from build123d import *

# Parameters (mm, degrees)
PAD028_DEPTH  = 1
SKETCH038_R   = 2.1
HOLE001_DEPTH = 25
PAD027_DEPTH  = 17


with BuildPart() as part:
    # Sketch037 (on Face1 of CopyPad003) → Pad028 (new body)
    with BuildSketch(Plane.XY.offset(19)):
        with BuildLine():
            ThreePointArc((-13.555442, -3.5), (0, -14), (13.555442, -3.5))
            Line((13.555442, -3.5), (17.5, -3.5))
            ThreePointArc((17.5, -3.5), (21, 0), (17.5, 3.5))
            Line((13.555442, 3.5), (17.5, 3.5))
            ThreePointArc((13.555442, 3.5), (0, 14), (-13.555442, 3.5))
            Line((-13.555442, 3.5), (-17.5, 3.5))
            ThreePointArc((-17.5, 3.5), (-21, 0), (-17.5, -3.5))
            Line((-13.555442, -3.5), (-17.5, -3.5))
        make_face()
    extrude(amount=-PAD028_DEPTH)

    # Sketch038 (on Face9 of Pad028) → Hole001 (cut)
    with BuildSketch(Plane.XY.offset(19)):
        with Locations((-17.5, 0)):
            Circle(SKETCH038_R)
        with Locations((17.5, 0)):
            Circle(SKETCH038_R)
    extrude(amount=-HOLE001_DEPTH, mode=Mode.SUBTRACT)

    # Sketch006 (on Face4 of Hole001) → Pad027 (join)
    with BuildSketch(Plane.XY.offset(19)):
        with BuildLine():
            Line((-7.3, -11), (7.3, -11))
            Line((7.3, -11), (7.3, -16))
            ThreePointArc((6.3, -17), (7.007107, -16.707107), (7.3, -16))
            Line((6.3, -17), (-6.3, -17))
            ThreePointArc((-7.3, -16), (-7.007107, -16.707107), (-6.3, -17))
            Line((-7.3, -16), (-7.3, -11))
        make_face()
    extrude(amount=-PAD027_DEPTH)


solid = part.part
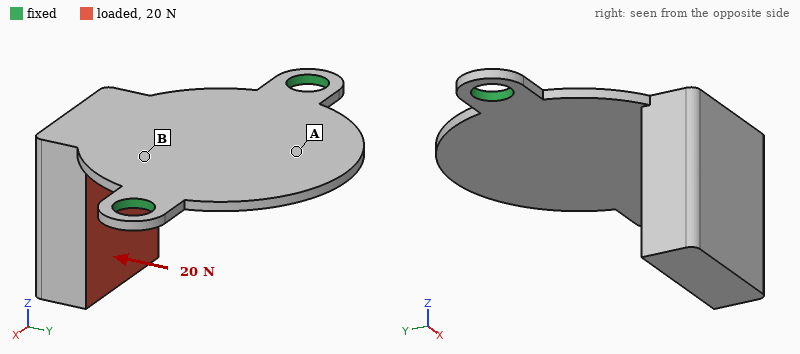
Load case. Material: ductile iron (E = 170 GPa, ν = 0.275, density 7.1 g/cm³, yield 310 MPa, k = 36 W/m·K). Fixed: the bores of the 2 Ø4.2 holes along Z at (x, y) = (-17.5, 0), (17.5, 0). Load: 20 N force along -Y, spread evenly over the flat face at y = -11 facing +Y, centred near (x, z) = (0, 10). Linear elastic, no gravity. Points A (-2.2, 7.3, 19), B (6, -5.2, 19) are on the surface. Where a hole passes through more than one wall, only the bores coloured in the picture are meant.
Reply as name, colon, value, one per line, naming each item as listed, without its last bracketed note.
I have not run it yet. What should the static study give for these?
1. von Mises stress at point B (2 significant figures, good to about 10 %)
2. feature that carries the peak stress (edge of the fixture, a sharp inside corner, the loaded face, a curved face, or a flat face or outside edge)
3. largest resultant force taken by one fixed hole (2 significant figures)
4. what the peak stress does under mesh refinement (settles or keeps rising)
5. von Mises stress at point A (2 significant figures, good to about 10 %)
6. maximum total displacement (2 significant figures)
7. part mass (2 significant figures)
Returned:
von Mises stress at point B: 36 MPa
feature that carries the peak stress: a sharp inside corner
largest resultant force taken by one fixed hole: 10 N
what the peak stress does under mesh refinement: keeps rising
von Mises stress at point A: 8.2 MPa
maximum total displacement: 0.16 mm
part mass: 15 g
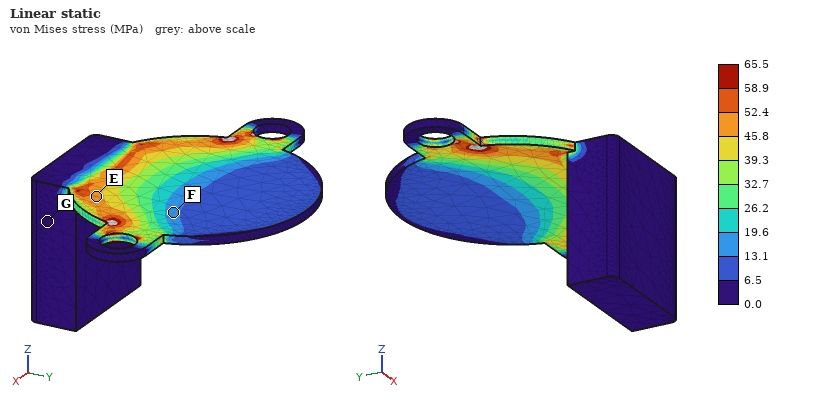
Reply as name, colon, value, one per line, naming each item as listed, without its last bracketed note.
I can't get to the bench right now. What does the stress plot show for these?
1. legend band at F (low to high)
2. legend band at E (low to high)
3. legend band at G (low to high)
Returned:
legend band at F: 13.1 to 19.6 MPa
legend band at E: 45.8 to 52.4 MPa
legend band at G: 0.0 to 6.5 MPa
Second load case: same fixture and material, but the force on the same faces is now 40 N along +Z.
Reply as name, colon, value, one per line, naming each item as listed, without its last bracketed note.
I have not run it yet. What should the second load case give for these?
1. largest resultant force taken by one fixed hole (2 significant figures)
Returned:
largest resultant force taken by one fixed hole: 20 N
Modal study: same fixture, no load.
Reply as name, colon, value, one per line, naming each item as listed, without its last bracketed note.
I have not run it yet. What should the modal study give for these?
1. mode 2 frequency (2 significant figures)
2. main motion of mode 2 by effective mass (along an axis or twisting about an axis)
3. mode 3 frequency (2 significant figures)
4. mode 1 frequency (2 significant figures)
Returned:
mode 2 frequency: 1500 Hz
main motion of mode 2 by effective mass: along X
mode 3 frequency: 1900 Hz
mode 1 frequency: 530 Hz
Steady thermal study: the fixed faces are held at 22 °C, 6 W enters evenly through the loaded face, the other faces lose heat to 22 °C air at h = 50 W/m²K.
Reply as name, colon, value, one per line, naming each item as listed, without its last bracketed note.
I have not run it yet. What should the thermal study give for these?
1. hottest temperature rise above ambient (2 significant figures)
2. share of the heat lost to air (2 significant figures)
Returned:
hottest temperature rise above ambient: 82 K
share of the heat lost to air: 67 %
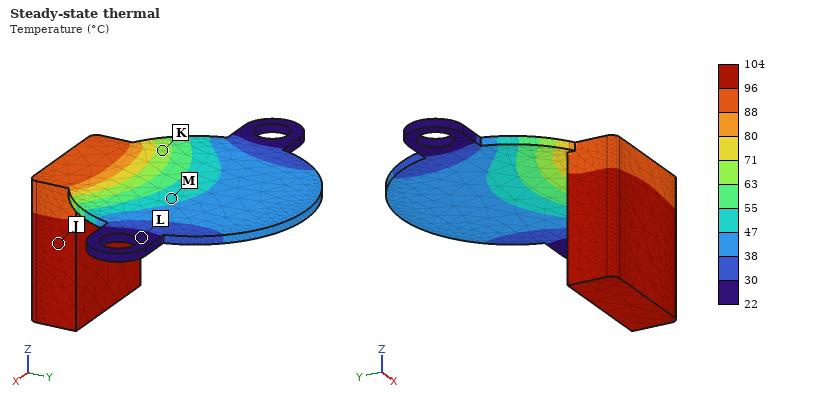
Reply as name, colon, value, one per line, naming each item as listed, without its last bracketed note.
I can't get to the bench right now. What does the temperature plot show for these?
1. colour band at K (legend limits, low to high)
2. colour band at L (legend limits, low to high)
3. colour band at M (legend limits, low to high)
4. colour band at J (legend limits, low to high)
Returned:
colour band at K: 63 to 71 °C
colour band at L: 22 to 30 °C
colour band at M: 47 to 55 °C
colour band at J: 96 to 104 °C
